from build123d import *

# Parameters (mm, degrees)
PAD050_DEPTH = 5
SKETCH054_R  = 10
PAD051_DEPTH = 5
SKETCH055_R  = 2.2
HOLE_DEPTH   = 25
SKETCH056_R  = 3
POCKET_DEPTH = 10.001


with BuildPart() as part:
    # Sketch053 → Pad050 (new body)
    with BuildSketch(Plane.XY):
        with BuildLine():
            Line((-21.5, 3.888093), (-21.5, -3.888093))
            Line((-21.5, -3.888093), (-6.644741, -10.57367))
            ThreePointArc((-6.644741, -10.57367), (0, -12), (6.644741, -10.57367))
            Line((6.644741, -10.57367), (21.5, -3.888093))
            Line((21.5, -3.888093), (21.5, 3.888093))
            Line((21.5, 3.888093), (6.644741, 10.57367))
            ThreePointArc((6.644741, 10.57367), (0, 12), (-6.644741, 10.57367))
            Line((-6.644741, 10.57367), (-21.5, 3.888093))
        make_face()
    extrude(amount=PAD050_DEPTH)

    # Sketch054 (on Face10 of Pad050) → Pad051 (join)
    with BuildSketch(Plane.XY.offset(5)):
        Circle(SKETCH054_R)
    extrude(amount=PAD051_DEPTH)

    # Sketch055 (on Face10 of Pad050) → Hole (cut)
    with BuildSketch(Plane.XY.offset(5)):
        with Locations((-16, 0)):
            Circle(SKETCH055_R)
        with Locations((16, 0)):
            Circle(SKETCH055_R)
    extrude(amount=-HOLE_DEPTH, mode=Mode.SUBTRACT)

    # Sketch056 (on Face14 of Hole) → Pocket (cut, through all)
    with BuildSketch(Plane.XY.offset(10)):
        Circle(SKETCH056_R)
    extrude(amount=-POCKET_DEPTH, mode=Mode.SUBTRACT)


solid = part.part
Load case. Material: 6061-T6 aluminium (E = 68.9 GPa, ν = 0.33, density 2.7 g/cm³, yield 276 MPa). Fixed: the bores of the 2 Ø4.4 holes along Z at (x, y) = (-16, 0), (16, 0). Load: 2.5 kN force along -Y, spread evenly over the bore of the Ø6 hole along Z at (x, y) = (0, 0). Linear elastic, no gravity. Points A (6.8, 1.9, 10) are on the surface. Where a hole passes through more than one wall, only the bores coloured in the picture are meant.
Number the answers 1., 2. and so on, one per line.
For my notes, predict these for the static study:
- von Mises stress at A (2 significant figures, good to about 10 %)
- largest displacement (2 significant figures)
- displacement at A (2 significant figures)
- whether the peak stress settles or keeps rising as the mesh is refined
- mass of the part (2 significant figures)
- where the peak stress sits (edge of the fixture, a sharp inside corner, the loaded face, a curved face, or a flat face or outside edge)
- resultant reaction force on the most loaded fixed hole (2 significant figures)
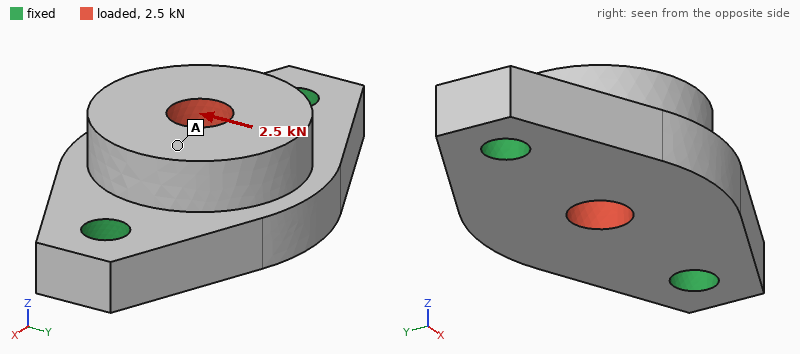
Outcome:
1. 9.6 MPa
2. 25 µm
3. 18 µm
4. keeps rising
5. 13 g
6. edge of the fixture
7. 1.3 kN
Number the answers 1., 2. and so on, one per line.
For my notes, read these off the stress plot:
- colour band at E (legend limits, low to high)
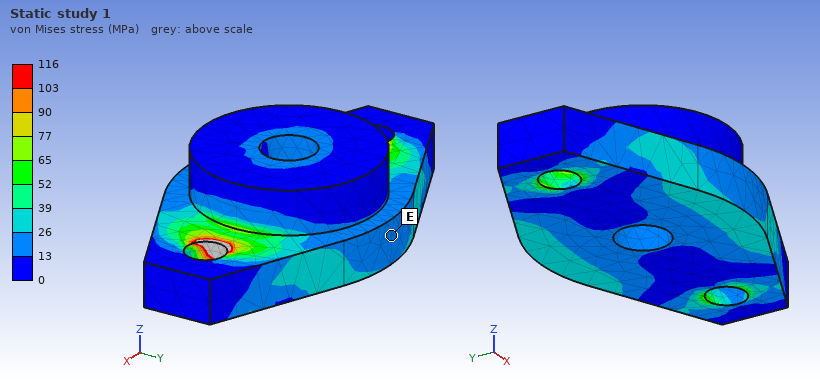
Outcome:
1. 13 to 26 MPa
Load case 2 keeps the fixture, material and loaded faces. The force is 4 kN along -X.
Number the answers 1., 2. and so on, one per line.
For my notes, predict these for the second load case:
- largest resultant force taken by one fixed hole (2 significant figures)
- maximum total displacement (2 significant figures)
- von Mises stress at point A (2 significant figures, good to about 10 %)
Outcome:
1. 2.0 kN
2. 8.2 µm
3. 14 MPa
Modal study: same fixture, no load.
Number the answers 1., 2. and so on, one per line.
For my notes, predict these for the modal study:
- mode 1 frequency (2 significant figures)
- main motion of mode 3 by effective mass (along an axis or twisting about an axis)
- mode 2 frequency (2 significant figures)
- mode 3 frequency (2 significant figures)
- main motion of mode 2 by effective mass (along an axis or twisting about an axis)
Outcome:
1. 15 kHz
2. along Y
3. 21 kHz
4. 32 kHz
5. along Z
